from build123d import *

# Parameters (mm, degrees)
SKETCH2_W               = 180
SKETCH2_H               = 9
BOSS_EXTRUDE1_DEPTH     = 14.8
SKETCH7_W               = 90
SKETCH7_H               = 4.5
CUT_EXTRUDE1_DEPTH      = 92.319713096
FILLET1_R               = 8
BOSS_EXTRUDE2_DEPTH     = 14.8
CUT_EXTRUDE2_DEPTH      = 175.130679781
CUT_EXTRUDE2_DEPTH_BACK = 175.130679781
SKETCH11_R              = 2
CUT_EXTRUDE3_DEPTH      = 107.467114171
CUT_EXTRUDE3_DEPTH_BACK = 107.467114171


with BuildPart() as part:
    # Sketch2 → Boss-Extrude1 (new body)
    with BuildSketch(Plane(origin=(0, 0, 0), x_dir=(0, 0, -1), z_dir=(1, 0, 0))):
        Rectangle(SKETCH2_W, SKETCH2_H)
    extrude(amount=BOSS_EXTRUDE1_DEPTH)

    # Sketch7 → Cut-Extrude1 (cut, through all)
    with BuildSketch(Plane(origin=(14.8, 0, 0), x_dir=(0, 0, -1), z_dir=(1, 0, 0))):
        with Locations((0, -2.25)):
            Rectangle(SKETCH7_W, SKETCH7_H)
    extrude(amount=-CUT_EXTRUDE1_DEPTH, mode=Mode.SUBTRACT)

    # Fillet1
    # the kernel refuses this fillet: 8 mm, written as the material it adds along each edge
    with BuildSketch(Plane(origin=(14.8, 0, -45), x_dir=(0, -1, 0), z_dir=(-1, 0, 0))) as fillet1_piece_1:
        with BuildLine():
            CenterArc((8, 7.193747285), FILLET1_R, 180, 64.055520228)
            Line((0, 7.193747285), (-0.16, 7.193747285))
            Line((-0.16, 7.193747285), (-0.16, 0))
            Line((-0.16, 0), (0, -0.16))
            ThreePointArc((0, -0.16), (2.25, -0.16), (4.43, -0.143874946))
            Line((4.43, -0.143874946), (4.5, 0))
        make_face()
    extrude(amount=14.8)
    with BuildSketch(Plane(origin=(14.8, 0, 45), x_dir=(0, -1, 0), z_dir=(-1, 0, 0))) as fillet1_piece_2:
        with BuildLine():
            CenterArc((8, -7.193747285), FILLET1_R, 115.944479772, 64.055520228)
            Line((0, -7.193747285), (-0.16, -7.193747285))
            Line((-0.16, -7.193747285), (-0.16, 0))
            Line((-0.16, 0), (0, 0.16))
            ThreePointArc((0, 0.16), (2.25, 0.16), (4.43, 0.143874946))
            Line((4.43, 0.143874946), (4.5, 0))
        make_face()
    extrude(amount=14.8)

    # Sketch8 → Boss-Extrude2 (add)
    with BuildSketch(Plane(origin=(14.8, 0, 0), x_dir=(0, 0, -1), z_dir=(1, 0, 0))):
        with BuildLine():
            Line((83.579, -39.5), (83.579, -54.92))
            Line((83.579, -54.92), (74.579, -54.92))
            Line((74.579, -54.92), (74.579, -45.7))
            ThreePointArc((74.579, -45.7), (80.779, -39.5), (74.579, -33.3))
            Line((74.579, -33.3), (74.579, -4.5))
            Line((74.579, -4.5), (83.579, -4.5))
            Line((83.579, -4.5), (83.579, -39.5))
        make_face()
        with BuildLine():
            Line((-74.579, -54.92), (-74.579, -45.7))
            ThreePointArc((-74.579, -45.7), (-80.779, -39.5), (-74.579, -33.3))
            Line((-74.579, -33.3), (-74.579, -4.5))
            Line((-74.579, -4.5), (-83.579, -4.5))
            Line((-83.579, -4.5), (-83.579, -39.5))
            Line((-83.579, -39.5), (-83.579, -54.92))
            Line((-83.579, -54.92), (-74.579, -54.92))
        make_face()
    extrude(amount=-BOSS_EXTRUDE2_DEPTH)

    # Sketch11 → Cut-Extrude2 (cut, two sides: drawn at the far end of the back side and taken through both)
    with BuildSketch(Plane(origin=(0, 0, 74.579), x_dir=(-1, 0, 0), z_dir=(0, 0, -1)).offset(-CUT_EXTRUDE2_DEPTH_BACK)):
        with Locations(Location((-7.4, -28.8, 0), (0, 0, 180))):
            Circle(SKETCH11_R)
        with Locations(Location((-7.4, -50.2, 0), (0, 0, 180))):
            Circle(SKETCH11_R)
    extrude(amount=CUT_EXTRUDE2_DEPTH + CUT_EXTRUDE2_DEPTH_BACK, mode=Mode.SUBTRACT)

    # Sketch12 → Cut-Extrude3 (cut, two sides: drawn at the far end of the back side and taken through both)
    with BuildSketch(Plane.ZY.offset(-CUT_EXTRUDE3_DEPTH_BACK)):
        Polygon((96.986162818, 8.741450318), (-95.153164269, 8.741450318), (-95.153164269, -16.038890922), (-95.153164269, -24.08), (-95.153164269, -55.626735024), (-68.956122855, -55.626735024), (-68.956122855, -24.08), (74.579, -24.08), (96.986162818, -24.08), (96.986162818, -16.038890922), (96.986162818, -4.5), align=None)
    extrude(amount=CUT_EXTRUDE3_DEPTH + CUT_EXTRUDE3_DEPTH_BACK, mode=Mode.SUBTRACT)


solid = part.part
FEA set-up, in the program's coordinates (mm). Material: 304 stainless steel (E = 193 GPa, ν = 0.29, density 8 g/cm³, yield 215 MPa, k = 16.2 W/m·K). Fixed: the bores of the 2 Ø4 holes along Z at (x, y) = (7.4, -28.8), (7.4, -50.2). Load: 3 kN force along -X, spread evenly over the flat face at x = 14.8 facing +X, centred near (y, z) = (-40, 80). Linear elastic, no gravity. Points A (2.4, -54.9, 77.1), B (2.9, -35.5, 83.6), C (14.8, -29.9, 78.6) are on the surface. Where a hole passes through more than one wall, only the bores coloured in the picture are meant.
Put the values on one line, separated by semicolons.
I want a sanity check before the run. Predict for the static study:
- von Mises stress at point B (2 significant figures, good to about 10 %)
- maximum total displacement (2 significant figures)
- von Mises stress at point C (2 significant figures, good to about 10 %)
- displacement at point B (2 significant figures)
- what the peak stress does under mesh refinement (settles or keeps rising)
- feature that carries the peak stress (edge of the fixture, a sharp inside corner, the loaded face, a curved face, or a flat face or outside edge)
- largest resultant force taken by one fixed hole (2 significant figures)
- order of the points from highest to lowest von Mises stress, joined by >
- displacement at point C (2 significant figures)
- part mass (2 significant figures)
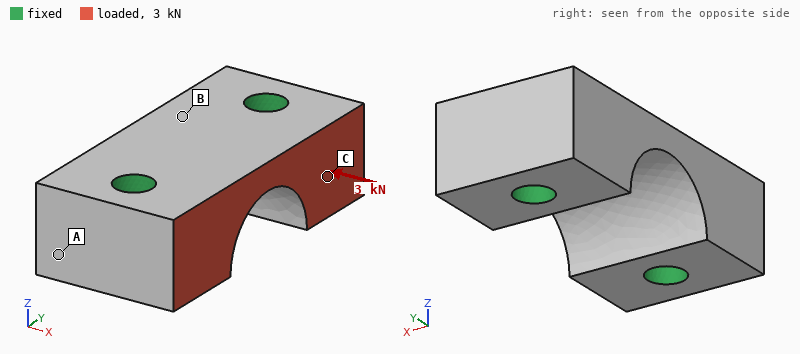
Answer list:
9.0 MPa; 1.4 µm; 18 MPa; 0.63 µm; keeps rising; edge of the fixture; 1.5 kN; C > B > A; 0.59 µm; 24 g
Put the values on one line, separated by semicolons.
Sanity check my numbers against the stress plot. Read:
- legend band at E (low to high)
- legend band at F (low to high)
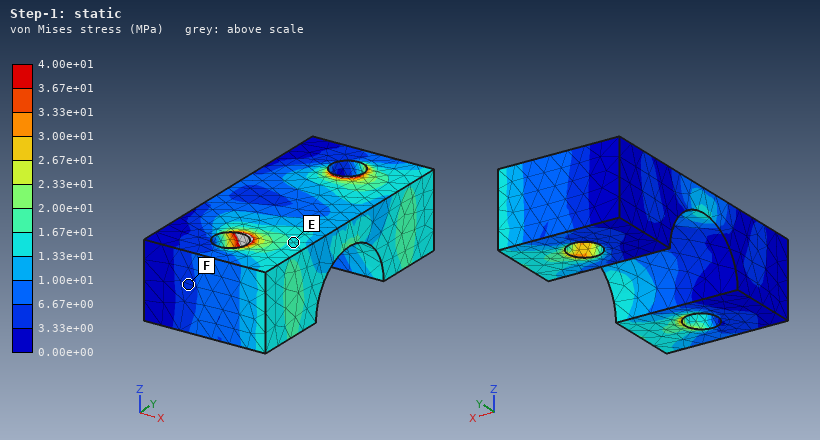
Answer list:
1.33e+01 to 1.67e+01 MPa; 3.33e+00 to 6.67e+00 MPa
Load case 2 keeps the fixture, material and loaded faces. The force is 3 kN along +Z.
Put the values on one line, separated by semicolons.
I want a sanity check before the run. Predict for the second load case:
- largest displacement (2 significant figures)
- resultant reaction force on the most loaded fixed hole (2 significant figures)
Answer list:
5.7 µm; 1.5 kN
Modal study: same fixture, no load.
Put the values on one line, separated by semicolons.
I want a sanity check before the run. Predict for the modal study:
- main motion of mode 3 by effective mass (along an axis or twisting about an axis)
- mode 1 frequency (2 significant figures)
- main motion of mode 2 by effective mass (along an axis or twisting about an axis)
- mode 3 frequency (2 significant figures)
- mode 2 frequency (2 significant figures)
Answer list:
twisting about Y; 55 kHz; along Z; 72 kHz; 63 kHz
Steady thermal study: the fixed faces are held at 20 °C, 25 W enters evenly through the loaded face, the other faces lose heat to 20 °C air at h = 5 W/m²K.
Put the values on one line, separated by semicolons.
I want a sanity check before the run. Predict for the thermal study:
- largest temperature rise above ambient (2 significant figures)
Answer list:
60 K
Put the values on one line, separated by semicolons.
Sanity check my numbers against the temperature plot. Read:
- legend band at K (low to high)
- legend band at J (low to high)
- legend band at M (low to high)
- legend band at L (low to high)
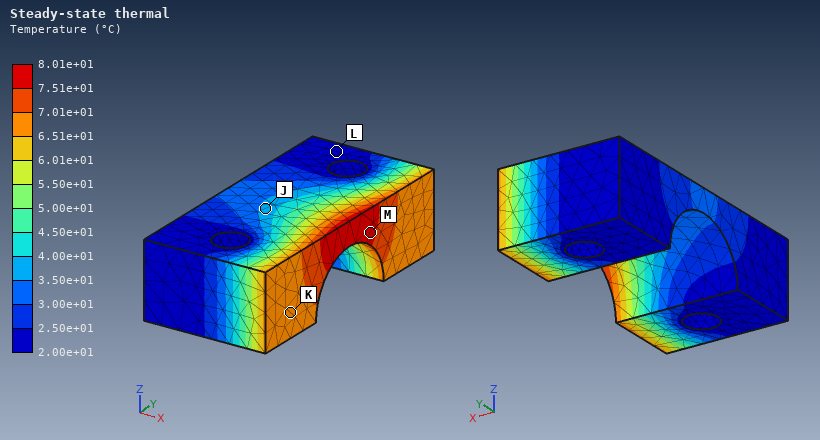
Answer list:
6.51e+01 to 7.01e+01 °C; 3.50e+01 to 4.00e+01 °C; 7.51e+01 to 8.01e+01 °C; 2.00e+01 to 2.50e+01 °C
